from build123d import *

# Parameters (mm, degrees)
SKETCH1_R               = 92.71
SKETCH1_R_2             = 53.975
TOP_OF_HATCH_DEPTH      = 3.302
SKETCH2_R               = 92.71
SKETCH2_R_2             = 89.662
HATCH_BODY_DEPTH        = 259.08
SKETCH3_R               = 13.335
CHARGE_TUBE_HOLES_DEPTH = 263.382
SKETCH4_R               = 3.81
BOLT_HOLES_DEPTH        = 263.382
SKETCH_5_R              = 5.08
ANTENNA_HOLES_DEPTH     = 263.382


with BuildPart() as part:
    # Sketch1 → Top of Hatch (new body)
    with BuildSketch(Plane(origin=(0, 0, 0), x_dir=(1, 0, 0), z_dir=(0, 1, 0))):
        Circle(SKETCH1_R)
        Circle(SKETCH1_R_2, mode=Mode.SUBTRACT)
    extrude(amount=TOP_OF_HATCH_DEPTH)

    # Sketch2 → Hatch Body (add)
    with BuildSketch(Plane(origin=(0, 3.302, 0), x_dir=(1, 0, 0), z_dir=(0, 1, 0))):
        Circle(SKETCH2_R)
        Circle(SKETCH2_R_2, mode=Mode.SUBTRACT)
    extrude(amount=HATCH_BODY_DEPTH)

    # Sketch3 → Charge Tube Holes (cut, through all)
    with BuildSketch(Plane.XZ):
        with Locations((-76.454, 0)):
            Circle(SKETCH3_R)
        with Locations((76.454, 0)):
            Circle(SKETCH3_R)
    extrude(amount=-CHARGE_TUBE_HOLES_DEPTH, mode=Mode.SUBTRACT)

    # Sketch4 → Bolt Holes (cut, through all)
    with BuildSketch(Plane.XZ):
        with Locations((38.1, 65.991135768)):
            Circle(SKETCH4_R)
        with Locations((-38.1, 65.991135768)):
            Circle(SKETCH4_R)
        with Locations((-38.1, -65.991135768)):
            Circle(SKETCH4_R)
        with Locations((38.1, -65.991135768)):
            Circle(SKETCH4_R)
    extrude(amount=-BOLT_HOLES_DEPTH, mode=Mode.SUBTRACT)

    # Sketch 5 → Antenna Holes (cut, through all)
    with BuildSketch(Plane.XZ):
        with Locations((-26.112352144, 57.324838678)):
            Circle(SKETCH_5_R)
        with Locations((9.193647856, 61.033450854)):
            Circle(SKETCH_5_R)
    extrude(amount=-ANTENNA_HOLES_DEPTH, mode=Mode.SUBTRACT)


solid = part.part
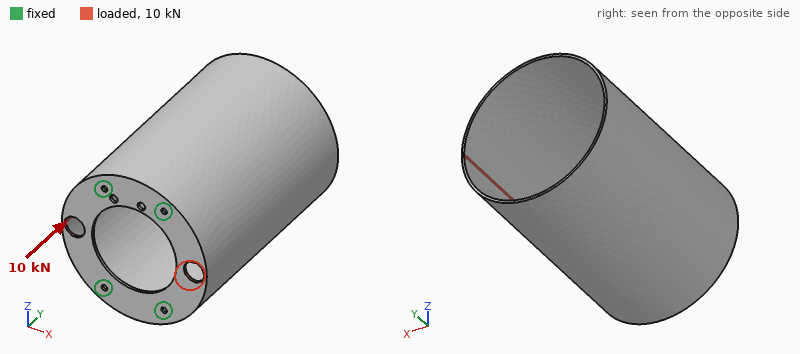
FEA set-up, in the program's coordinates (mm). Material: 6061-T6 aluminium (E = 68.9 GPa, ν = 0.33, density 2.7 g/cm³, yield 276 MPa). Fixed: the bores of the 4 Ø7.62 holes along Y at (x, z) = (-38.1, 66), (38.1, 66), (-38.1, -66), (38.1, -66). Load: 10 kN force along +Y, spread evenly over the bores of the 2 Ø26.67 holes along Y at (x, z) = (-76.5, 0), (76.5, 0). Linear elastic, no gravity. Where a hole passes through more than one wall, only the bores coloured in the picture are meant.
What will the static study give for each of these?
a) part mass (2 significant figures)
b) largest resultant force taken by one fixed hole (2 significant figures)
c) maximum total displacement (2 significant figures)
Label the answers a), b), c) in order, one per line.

a) 1.4 kg
b) 2.8 kN
c) 1.7 mm
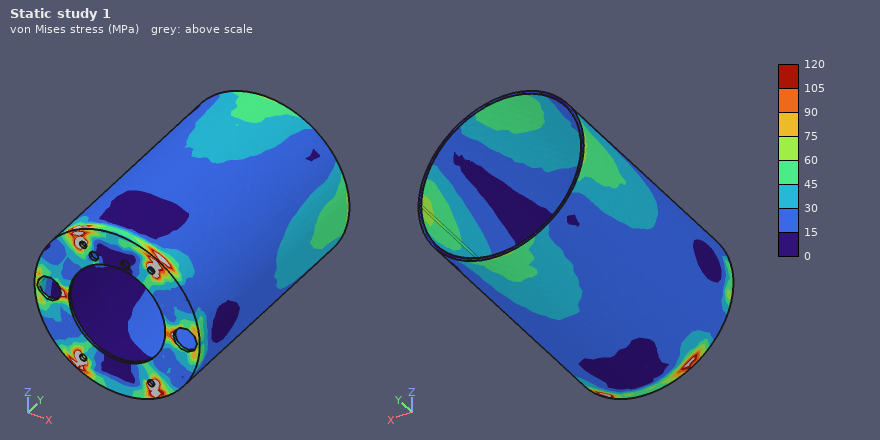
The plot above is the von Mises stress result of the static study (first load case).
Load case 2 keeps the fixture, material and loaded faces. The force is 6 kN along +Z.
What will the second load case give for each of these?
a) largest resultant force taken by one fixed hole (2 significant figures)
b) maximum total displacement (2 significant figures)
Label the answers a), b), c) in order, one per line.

a) 2.9 kN
b) 0.64 mm
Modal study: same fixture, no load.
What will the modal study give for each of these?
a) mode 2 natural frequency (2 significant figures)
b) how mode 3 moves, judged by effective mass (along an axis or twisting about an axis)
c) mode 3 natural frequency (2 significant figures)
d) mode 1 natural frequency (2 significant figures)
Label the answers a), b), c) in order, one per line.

a) 300 Hz
b) along X
c) 310 Hz
d) 260 Hz
